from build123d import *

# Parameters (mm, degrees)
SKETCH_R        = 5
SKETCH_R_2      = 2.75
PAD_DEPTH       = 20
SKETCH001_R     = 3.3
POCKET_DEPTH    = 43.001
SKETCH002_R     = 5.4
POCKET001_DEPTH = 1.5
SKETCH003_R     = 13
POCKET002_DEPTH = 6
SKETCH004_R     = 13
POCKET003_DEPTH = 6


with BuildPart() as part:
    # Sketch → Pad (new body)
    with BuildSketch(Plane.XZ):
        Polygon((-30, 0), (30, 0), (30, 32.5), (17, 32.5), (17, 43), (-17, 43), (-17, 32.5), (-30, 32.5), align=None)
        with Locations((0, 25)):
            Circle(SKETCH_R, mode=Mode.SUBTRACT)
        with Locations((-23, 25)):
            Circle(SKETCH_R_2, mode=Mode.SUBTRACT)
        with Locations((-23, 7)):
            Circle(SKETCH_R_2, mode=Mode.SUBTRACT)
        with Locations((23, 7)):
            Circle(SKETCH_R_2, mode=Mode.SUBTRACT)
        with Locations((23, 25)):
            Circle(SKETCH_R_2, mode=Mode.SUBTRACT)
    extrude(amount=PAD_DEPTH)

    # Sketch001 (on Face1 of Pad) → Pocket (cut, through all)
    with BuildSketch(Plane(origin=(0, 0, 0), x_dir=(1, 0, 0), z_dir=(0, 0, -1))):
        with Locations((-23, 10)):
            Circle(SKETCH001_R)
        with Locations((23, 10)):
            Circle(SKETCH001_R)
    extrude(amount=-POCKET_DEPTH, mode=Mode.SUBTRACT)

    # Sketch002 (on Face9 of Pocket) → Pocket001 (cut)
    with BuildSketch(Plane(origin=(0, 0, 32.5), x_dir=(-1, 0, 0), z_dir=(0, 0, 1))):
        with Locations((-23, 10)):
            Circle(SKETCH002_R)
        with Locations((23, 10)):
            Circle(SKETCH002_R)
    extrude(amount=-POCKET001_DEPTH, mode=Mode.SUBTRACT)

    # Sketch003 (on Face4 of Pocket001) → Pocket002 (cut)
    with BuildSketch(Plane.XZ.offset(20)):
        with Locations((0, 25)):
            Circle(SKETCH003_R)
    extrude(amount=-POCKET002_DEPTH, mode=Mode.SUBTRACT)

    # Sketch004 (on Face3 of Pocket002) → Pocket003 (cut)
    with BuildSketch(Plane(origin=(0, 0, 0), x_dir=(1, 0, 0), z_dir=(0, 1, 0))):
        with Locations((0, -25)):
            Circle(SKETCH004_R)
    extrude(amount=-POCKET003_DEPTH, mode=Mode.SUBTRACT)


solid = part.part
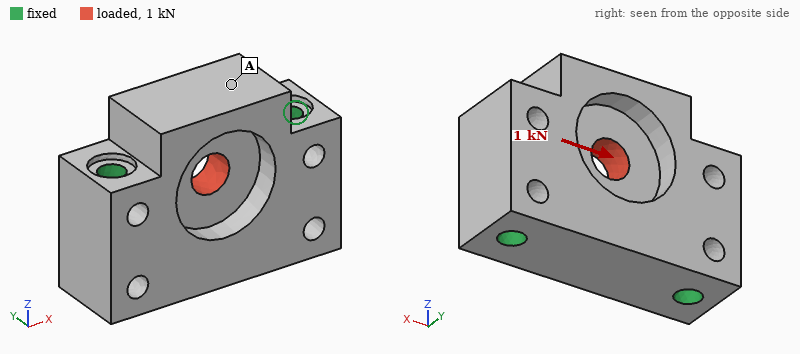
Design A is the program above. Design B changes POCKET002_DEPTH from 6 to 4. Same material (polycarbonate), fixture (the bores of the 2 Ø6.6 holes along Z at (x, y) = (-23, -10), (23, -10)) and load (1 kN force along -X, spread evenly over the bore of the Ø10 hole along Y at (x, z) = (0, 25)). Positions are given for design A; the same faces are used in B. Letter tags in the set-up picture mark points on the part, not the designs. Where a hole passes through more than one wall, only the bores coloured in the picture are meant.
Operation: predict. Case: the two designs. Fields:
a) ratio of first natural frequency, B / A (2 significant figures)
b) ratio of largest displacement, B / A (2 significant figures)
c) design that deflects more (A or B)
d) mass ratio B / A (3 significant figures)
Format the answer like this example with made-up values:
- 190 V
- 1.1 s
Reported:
- 1.0
- 0.87
- A
- 1.03
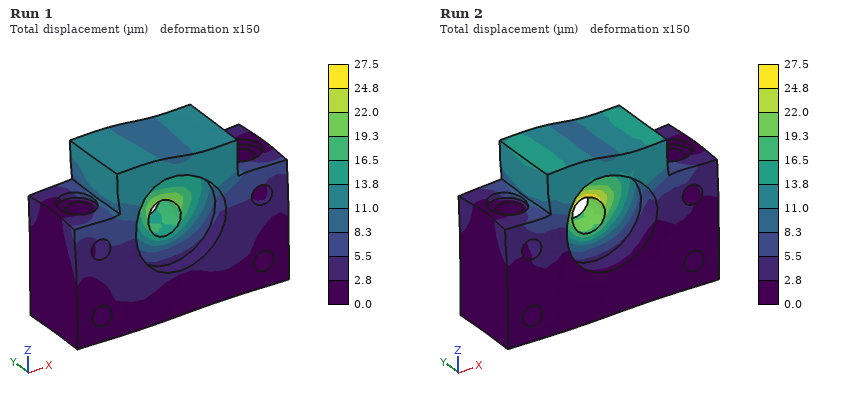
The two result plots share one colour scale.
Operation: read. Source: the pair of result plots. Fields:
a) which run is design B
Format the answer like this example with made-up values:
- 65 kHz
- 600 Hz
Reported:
- Run 1
